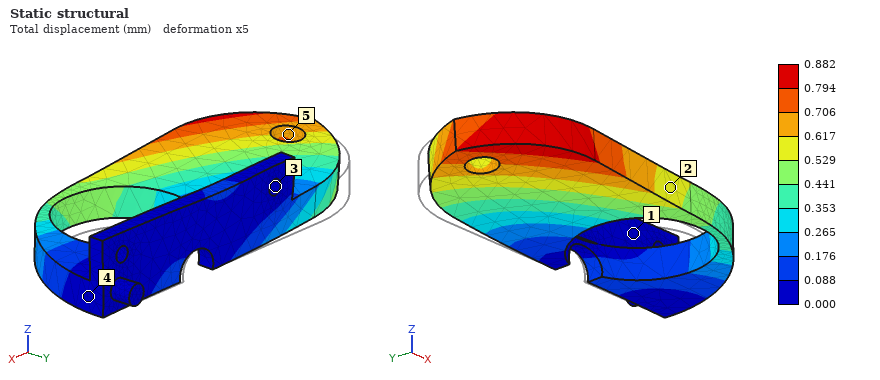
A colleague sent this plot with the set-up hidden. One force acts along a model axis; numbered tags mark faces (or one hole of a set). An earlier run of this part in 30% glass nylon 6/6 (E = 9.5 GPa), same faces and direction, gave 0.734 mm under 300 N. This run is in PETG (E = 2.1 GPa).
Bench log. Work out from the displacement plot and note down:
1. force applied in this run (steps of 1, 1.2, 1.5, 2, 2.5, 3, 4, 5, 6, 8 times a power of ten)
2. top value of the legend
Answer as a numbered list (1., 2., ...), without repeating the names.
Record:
1. 80 N
2. 0.882 mm
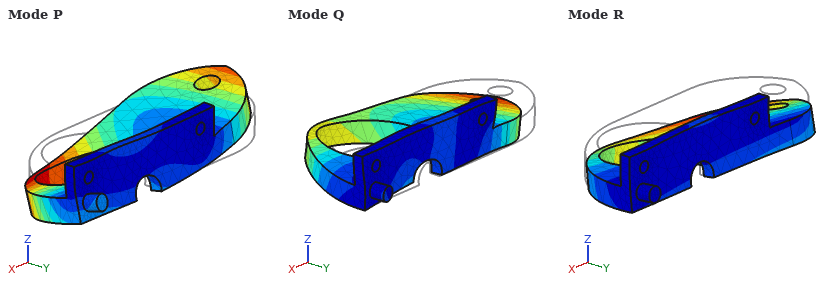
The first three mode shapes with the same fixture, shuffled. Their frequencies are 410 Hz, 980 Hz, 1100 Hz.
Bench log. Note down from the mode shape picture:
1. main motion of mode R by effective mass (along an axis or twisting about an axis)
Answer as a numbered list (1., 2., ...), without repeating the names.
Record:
1. along Z
